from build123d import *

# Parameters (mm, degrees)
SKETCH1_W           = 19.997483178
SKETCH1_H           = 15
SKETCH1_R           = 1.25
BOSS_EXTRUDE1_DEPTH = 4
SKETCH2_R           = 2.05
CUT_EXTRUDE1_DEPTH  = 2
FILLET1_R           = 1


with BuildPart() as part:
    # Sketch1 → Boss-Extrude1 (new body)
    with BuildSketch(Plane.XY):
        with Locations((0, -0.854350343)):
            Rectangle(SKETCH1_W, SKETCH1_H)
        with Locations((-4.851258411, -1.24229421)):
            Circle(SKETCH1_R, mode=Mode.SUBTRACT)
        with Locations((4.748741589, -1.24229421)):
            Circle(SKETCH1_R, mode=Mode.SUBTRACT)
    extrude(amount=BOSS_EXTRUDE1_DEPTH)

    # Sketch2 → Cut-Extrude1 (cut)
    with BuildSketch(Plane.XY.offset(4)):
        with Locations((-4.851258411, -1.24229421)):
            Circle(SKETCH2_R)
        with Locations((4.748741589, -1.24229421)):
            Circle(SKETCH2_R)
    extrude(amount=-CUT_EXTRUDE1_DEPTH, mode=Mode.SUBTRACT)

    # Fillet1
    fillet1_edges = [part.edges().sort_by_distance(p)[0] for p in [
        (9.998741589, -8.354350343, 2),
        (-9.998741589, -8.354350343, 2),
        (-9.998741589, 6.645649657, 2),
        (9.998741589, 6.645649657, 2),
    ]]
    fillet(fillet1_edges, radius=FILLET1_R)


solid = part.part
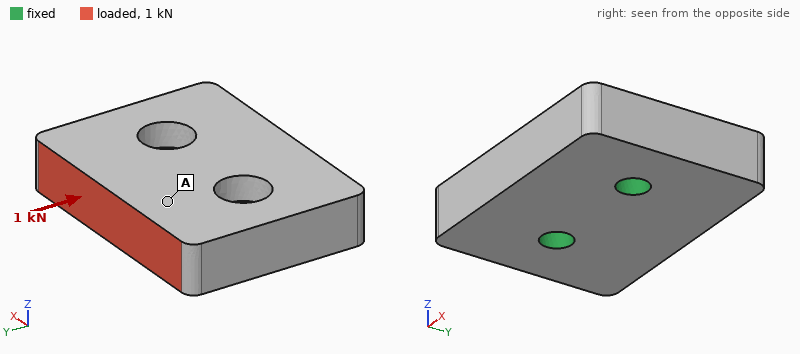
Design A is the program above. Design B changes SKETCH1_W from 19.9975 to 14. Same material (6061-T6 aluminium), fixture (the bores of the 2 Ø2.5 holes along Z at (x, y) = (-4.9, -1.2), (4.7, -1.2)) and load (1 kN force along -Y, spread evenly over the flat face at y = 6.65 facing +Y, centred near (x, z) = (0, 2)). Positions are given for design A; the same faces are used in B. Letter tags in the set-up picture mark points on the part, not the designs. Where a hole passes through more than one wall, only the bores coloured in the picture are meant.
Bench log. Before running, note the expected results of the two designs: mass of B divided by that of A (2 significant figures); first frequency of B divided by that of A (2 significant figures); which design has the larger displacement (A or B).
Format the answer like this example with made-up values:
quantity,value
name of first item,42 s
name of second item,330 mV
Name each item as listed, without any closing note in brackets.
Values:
quantity,value
mass of B divided by that of A,0.68
first frequency of B divided by that of A,1.1
which design has the larger displacement,B
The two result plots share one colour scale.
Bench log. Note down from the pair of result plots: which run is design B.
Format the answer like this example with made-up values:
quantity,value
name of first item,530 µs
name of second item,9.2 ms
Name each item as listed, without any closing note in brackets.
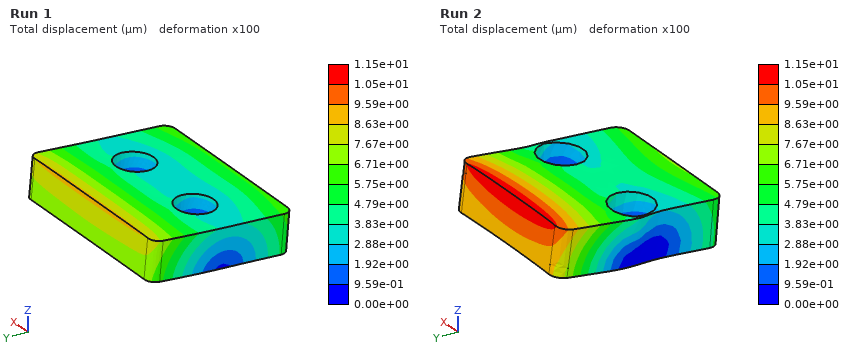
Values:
quantity,value
which run is design B,Run 2
